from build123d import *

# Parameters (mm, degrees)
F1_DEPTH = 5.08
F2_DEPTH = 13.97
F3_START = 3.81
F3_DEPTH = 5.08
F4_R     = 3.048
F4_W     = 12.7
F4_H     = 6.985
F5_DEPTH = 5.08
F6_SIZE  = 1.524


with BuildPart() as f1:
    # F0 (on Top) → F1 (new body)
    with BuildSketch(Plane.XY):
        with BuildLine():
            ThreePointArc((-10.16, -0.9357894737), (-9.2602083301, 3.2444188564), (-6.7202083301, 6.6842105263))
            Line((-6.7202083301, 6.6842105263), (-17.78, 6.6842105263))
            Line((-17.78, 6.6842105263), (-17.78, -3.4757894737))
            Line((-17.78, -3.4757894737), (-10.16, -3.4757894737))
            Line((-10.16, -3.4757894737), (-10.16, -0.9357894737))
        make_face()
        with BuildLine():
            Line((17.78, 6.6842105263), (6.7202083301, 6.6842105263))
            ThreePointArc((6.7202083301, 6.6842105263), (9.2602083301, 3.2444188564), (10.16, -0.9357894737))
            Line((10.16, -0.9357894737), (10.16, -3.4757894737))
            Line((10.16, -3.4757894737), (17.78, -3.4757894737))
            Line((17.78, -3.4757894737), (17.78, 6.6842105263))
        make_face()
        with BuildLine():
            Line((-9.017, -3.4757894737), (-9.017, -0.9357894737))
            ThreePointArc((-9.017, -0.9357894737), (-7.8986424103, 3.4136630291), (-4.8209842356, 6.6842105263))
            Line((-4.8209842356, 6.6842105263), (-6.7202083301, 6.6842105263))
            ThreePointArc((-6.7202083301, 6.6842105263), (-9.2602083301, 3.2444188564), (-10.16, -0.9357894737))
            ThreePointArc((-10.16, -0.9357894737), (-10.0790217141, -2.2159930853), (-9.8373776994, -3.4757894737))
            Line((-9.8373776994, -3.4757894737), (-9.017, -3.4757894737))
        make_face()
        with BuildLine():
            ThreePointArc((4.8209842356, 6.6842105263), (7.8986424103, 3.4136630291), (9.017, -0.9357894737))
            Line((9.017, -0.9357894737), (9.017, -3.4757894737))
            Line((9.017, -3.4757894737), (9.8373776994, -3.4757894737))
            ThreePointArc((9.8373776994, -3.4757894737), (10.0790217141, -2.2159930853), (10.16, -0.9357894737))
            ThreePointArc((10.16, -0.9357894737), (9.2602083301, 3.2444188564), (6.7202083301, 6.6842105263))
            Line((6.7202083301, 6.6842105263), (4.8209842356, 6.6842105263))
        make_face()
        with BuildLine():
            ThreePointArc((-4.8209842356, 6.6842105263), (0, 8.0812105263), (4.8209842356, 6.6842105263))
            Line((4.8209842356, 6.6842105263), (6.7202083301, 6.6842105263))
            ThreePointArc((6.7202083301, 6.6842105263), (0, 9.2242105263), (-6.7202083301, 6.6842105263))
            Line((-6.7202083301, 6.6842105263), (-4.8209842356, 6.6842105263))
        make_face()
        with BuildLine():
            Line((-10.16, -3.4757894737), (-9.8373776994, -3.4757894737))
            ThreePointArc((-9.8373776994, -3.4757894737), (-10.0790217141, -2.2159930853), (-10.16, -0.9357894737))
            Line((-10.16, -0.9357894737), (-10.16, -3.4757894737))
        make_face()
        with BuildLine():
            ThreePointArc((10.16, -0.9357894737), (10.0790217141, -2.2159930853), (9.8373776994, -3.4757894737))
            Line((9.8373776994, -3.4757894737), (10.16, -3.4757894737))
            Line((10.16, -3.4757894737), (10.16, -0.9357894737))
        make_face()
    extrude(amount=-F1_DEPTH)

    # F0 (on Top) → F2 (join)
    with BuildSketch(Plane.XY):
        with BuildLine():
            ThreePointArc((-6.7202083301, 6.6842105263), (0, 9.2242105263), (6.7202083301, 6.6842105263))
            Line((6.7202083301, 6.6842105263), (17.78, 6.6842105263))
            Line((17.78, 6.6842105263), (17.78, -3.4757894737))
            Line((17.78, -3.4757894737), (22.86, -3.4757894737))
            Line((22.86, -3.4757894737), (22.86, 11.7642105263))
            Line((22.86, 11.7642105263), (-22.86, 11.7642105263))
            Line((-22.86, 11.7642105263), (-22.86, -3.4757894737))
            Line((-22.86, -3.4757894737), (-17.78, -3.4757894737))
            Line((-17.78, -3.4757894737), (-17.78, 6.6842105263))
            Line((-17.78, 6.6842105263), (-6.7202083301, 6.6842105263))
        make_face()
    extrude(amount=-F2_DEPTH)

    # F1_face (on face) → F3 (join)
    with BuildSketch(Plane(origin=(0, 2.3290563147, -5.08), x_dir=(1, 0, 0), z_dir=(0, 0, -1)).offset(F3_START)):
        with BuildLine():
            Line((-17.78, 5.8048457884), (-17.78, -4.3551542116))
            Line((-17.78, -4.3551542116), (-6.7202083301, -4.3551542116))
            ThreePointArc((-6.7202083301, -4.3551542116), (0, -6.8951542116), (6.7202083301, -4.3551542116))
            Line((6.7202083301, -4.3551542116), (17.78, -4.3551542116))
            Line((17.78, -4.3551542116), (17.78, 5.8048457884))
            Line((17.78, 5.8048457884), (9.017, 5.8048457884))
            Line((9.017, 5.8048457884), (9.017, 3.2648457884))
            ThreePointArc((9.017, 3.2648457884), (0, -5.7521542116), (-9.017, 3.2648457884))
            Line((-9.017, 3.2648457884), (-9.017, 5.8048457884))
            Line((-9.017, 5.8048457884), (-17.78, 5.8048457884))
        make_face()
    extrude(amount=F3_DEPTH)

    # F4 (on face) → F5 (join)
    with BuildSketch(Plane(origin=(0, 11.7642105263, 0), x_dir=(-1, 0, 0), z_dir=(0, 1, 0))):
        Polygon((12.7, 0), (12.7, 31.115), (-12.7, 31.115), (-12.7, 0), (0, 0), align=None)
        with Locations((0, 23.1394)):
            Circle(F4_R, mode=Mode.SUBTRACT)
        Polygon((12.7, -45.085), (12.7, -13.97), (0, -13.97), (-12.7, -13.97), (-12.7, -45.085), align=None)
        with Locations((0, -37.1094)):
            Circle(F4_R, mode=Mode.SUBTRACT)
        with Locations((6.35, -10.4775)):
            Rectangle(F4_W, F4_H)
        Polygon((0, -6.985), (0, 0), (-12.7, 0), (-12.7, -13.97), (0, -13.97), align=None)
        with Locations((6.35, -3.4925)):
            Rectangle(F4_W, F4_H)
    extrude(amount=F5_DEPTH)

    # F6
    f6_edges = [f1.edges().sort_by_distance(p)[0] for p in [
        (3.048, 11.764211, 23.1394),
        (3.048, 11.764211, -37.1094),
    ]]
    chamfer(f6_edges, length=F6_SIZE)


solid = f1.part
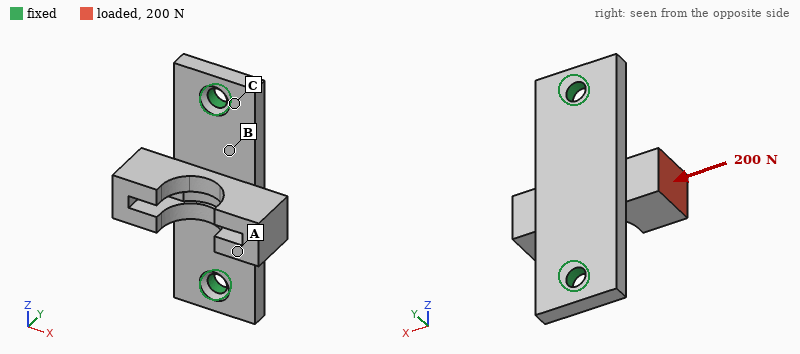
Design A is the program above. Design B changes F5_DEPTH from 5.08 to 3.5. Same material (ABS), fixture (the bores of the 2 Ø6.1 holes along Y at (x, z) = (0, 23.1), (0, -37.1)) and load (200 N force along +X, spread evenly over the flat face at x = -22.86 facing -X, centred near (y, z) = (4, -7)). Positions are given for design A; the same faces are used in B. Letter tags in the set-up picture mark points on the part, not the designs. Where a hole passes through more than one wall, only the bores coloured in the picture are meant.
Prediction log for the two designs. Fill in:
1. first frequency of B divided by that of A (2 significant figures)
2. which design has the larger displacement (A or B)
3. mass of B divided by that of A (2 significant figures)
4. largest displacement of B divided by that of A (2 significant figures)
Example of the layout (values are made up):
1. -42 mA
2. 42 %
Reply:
1. 0.62
2. B
3. 0.81
4. 2.3
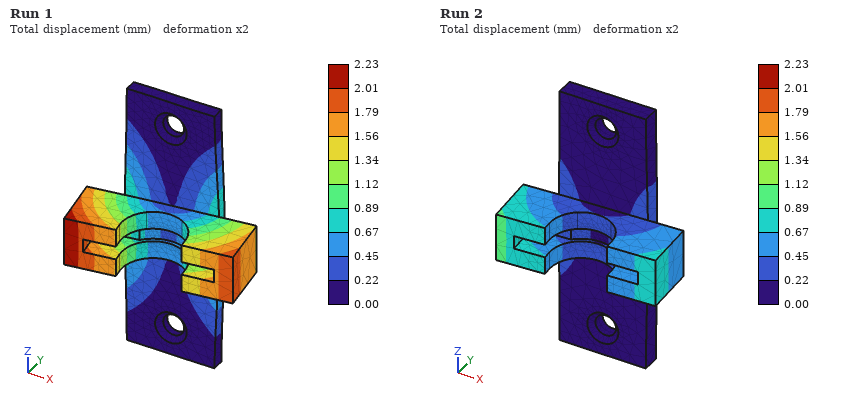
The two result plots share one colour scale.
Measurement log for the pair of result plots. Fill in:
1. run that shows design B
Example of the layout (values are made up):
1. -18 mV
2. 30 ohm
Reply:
1. Run 1
